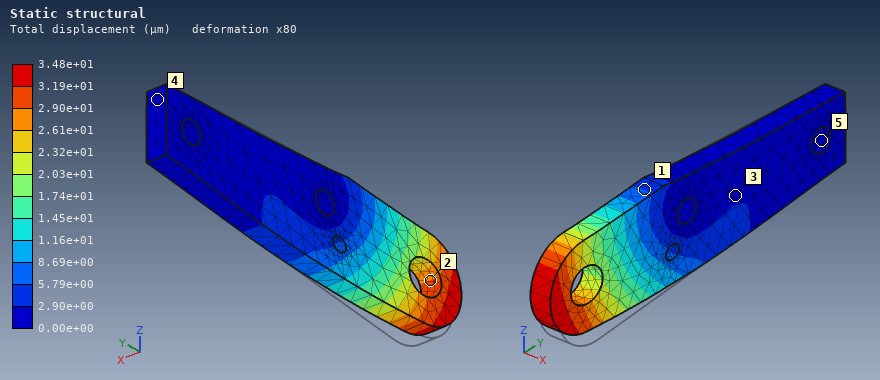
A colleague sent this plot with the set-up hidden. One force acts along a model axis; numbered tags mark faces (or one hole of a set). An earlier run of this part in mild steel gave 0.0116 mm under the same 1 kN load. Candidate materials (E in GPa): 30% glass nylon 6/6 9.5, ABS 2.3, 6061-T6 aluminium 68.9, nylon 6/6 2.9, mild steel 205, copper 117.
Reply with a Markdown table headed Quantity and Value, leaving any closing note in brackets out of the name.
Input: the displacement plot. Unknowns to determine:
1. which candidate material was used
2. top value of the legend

| Quantity | Value |
|---|---|
| which candidate material was used | 6061-T6 aluminium |
| top value of the legend | 3.48e+01 µm |
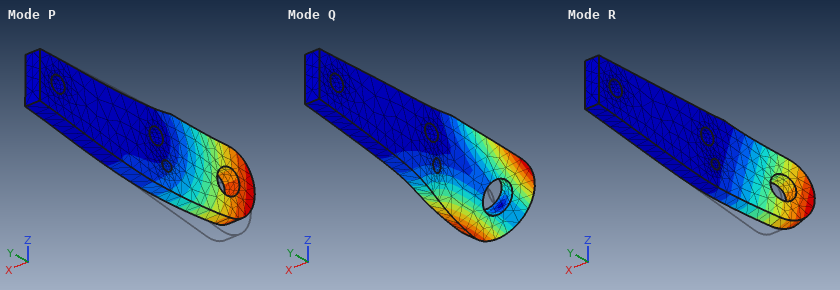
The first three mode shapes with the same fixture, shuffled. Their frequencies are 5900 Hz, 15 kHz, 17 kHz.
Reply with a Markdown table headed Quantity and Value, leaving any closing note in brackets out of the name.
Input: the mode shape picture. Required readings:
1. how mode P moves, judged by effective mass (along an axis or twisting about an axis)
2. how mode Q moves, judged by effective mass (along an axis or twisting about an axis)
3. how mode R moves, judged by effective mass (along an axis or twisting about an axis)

| Quantity | Value |
|---|---|
| how mode P moves, judged by effective mass | along Z |
| how mode Q moves, judged by effective mass | twisting about Y |
| how mode R moves, judged by effective mass | along X |
